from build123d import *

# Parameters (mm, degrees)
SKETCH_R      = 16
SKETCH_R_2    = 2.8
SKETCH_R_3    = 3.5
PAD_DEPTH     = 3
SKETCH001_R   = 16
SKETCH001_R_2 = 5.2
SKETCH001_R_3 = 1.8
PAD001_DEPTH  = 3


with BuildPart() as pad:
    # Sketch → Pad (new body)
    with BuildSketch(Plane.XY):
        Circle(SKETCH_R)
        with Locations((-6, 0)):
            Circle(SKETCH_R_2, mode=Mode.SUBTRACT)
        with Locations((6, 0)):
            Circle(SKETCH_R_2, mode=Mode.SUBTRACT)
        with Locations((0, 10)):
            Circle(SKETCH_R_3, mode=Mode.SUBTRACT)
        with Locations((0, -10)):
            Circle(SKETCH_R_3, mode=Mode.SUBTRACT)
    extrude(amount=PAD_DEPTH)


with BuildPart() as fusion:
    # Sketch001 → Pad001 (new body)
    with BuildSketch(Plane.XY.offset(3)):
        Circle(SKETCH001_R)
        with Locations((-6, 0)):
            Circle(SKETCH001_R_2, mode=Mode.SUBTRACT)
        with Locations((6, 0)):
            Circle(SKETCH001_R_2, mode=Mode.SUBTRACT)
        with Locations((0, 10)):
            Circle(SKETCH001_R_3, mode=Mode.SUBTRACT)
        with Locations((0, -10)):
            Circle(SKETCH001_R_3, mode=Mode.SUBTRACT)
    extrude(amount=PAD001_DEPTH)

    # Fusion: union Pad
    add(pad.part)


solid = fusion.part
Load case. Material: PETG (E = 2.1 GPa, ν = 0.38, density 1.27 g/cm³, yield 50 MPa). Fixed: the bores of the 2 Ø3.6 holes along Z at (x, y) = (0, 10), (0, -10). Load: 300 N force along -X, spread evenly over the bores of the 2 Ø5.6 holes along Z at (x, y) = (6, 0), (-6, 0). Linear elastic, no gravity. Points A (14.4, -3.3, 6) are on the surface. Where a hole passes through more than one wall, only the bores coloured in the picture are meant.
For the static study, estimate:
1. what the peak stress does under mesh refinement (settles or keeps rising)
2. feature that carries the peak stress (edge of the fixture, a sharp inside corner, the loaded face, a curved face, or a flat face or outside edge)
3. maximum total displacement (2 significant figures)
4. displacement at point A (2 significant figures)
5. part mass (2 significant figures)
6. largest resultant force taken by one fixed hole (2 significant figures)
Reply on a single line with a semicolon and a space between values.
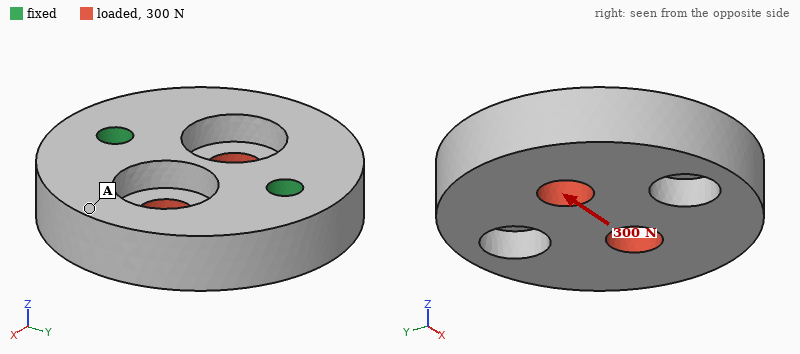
keeps rising; edge of the fixture; 0.16 mm; 0.13 mm; 4.9 g; 150 N
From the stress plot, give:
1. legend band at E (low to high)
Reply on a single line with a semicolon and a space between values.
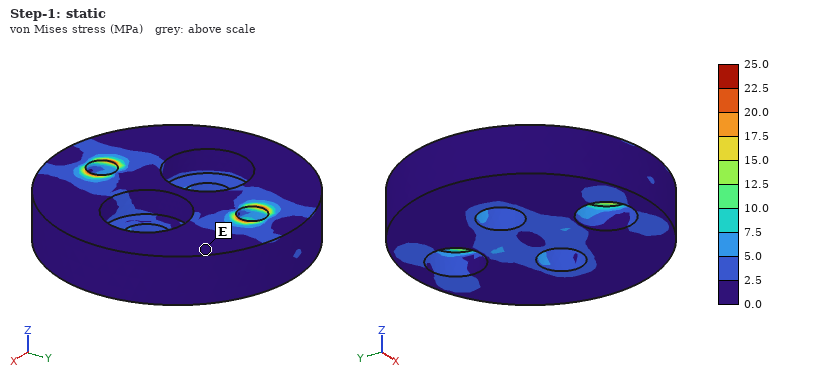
0.0 to 2.5 MPa
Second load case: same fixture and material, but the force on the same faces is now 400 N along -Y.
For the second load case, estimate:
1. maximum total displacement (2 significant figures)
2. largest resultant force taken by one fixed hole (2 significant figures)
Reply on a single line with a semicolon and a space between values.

36 µm; 210 N
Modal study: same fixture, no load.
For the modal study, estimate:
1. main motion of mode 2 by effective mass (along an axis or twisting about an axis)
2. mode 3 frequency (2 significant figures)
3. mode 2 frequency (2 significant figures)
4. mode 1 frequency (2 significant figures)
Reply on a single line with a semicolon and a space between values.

along Z; 6300 Hz; 4400 Hz; 2700 Hz
